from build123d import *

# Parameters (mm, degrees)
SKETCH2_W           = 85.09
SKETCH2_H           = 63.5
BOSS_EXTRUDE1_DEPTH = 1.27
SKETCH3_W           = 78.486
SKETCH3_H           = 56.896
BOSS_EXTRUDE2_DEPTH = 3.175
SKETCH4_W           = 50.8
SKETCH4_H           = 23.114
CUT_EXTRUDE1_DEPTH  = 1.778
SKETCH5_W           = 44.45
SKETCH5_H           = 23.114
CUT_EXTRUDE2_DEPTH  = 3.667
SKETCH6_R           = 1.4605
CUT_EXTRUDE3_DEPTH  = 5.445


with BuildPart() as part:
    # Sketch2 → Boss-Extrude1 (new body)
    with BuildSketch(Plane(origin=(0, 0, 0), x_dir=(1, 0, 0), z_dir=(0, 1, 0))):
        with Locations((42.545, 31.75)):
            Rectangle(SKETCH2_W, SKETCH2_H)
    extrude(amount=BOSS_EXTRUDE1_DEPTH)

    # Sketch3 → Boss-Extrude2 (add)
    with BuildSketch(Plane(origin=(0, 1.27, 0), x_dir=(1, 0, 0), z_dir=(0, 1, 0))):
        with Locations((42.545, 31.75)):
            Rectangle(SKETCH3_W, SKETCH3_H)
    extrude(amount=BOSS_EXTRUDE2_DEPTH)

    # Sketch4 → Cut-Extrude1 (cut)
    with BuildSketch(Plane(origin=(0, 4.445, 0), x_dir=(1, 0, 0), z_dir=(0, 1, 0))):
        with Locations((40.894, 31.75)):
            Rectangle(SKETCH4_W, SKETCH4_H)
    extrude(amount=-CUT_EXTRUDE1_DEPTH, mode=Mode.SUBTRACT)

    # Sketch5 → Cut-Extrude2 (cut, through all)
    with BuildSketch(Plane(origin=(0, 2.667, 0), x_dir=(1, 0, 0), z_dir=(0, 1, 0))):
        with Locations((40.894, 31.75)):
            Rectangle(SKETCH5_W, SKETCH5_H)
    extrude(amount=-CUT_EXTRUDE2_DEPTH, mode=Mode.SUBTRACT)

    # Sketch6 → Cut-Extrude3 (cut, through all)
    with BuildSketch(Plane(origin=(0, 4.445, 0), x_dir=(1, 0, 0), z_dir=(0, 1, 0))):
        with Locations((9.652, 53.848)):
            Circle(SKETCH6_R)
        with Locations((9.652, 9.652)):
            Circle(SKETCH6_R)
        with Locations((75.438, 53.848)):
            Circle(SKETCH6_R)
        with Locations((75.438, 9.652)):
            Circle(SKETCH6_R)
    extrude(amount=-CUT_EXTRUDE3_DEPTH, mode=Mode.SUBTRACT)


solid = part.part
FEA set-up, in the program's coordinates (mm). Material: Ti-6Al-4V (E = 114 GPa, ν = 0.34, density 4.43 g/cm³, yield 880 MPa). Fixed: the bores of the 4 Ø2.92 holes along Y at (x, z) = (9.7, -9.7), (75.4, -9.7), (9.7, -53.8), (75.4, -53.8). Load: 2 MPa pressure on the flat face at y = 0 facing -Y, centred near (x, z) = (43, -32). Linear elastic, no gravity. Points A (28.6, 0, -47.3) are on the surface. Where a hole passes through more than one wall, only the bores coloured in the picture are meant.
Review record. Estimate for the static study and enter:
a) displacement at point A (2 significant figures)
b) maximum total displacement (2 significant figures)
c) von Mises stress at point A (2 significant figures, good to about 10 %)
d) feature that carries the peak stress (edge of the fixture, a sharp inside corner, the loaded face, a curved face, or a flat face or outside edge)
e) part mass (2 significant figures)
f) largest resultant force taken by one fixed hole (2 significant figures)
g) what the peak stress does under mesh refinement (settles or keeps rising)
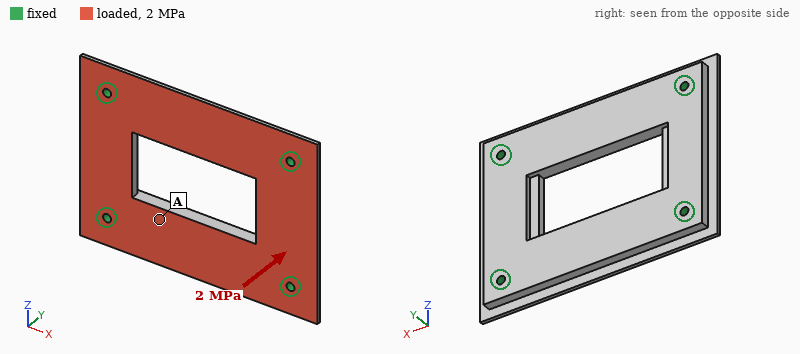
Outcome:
0.11 mm
0.16 mm
57 MPa
edge of the fixture
71 g
2.2 kN
keeps rising
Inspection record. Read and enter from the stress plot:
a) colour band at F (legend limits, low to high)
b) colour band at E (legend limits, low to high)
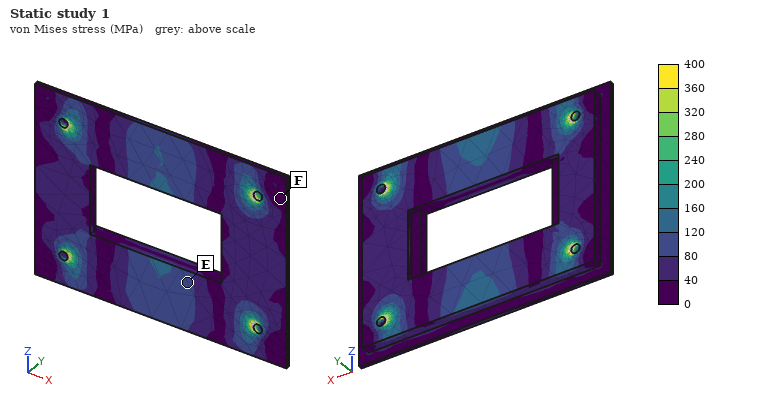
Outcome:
0 to 40 MPa
80 to 120 MPa
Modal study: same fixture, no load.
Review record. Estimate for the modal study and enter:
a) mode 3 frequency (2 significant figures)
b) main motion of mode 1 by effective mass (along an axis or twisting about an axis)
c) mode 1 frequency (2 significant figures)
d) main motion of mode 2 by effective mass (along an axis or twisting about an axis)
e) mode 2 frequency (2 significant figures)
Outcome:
8900 Hz
along Y
4900 Hz
twisting about X
5300 Hz
